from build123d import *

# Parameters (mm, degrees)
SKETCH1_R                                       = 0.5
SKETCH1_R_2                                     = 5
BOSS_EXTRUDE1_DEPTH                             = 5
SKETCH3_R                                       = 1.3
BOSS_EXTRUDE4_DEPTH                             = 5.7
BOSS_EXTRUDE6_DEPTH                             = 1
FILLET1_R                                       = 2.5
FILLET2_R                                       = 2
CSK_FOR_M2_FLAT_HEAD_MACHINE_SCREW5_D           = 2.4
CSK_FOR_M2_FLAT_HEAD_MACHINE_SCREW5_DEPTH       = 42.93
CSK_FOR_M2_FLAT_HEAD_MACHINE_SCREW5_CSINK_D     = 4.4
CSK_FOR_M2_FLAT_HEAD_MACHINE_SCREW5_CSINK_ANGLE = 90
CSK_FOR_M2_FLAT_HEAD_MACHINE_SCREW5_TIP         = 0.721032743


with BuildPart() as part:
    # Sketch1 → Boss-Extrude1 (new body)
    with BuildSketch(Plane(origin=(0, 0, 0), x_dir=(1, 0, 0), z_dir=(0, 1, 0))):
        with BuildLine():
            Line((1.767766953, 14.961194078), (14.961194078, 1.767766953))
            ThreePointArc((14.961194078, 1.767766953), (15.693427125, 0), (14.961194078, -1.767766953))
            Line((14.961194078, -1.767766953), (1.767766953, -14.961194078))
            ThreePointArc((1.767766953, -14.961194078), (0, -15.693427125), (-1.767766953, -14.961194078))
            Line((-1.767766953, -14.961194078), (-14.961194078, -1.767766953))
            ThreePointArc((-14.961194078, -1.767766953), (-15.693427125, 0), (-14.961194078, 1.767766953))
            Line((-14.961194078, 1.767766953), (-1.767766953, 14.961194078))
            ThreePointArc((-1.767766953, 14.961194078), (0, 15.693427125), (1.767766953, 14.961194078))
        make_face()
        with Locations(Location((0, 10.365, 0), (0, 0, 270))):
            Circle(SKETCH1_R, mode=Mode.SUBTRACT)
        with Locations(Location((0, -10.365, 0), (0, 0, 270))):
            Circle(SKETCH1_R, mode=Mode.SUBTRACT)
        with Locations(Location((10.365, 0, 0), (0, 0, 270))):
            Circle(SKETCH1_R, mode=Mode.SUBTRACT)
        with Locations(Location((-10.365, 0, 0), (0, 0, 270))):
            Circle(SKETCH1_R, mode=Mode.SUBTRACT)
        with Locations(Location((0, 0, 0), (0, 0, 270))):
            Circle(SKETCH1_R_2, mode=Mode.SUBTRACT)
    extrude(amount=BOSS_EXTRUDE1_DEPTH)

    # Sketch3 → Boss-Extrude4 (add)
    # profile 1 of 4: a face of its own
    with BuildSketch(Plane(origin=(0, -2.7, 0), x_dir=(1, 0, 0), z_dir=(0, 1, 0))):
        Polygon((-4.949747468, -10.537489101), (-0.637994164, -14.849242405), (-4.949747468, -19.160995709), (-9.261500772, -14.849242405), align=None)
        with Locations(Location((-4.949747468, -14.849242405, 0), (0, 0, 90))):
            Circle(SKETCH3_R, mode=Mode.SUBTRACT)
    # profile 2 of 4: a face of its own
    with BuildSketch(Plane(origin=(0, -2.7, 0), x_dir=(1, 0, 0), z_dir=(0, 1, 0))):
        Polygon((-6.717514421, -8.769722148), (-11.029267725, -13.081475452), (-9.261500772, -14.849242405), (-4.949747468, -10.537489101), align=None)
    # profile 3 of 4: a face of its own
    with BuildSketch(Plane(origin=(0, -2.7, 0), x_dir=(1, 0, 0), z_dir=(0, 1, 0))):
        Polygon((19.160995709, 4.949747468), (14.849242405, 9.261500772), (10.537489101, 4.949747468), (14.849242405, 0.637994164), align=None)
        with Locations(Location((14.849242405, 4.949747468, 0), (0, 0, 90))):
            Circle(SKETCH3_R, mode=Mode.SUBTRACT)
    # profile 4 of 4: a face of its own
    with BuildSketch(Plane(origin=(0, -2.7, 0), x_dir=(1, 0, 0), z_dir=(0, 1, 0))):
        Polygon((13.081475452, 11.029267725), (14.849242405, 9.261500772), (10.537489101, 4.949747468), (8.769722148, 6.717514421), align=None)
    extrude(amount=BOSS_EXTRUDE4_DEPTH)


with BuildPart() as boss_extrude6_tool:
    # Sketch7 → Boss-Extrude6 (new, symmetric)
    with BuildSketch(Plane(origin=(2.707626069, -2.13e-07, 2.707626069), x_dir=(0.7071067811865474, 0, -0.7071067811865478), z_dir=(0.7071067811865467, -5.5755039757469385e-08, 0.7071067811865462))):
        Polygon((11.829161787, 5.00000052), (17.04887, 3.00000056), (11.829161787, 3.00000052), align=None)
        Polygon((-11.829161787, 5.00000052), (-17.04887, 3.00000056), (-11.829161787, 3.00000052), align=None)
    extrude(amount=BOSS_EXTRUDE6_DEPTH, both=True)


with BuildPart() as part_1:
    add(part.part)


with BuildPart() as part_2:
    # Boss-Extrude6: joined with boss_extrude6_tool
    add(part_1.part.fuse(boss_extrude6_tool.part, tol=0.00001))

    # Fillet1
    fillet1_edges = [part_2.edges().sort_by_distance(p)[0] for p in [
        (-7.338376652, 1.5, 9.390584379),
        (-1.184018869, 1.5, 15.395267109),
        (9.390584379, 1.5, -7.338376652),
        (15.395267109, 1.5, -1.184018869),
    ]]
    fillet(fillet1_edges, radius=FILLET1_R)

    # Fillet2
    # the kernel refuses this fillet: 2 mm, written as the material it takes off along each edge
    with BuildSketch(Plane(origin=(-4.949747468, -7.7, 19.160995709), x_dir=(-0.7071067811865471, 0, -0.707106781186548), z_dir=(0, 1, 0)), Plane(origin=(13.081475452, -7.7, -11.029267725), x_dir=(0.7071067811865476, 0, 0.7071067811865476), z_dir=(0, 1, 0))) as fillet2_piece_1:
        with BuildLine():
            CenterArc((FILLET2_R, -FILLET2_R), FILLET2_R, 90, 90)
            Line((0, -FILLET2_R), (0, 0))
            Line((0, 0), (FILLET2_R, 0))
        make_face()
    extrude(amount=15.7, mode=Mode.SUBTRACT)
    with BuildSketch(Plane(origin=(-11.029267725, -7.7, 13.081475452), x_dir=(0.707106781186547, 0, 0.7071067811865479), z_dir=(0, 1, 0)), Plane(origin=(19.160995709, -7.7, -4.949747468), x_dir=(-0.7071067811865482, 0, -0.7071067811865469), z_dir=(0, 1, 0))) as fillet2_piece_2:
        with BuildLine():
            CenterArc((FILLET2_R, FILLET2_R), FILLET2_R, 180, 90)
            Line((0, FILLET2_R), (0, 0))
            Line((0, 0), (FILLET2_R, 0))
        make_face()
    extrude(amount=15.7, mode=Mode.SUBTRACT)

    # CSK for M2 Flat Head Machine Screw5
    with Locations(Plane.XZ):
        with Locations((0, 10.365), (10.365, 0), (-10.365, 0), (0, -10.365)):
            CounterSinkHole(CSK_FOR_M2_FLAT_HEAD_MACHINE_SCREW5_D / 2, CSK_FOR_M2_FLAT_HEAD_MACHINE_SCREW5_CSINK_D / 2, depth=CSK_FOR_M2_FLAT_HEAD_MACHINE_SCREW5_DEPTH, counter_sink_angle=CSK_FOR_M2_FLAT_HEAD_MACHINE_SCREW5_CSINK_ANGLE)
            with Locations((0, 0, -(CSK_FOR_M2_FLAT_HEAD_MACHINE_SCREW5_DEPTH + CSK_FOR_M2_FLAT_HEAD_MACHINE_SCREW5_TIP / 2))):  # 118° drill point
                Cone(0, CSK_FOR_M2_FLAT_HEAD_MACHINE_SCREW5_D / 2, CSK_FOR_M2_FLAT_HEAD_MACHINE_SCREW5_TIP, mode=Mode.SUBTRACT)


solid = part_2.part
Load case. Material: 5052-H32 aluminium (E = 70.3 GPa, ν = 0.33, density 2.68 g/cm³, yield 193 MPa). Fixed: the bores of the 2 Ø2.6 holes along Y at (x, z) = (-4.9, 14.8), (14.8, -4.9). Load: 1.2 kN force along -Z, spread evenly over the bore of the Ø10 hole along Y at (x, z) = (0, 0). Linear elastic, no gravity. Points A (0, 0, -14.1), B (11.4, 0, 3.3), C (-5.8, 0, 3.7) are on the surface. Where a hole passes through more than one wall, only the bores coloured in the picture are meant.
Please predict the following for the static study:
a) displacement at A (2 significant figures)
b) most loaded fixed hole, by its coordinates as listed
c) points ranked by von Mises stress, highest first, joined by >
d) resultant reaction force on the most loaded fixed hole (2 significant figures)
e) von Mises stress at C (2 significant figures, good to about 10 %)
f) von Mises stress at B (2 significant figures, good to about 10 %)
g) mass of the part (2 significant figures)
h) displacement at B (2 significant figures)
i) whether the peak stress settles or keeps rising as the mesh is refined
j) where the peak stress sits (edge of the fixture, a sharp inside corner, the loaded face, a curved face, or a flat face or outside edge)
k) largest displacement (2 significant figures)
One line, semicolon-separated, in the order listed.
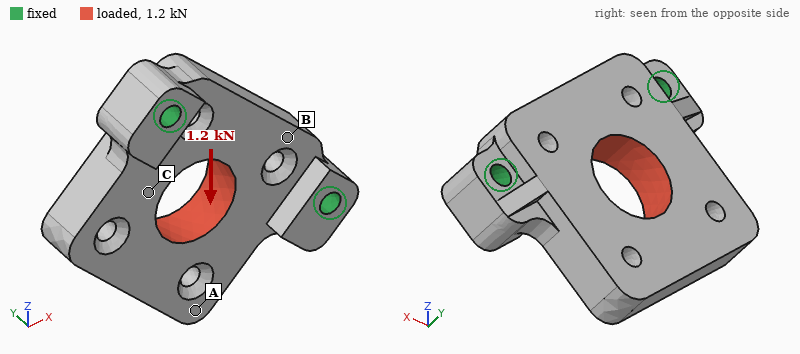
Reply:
8.7 µm; (-4.9, 14.8); C > B > A; 790 N; 32 MPa; 19 MPa; 7.4 g; 3.8 µm; keeps rising; edge of the fixture; 12 µm
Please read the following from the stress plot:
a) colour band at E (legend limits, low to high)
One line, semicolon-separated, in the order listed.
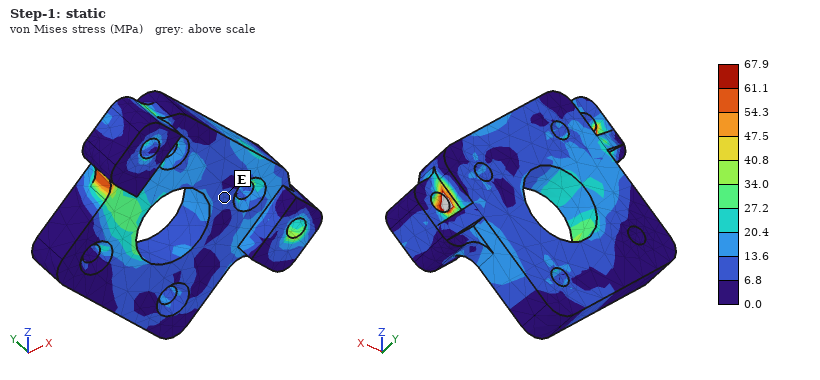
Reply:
6.8 to 13.6 MPa
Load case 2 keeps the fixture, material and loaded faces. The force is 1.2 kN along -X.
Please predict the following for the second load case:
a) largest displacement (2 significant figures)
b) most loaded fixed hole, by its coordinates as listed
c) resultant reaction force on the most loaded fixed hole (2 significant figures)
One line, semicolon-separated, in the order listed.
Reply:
12 µm; (14.8, -4.9); 790 N
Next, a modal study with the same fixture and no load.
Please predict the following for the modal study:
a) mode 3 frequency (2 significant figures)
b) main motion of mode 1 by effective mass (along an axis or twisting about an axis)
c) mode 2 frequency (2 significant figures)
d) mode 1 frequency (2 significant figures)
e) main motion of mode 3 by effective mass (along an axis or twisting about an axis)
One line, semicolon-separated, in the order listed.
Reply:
27 kHz; along Y; 20 kHz; 8500 Hz; along Y
